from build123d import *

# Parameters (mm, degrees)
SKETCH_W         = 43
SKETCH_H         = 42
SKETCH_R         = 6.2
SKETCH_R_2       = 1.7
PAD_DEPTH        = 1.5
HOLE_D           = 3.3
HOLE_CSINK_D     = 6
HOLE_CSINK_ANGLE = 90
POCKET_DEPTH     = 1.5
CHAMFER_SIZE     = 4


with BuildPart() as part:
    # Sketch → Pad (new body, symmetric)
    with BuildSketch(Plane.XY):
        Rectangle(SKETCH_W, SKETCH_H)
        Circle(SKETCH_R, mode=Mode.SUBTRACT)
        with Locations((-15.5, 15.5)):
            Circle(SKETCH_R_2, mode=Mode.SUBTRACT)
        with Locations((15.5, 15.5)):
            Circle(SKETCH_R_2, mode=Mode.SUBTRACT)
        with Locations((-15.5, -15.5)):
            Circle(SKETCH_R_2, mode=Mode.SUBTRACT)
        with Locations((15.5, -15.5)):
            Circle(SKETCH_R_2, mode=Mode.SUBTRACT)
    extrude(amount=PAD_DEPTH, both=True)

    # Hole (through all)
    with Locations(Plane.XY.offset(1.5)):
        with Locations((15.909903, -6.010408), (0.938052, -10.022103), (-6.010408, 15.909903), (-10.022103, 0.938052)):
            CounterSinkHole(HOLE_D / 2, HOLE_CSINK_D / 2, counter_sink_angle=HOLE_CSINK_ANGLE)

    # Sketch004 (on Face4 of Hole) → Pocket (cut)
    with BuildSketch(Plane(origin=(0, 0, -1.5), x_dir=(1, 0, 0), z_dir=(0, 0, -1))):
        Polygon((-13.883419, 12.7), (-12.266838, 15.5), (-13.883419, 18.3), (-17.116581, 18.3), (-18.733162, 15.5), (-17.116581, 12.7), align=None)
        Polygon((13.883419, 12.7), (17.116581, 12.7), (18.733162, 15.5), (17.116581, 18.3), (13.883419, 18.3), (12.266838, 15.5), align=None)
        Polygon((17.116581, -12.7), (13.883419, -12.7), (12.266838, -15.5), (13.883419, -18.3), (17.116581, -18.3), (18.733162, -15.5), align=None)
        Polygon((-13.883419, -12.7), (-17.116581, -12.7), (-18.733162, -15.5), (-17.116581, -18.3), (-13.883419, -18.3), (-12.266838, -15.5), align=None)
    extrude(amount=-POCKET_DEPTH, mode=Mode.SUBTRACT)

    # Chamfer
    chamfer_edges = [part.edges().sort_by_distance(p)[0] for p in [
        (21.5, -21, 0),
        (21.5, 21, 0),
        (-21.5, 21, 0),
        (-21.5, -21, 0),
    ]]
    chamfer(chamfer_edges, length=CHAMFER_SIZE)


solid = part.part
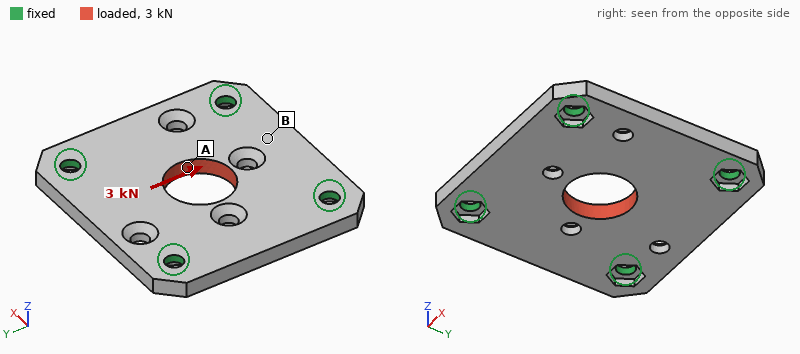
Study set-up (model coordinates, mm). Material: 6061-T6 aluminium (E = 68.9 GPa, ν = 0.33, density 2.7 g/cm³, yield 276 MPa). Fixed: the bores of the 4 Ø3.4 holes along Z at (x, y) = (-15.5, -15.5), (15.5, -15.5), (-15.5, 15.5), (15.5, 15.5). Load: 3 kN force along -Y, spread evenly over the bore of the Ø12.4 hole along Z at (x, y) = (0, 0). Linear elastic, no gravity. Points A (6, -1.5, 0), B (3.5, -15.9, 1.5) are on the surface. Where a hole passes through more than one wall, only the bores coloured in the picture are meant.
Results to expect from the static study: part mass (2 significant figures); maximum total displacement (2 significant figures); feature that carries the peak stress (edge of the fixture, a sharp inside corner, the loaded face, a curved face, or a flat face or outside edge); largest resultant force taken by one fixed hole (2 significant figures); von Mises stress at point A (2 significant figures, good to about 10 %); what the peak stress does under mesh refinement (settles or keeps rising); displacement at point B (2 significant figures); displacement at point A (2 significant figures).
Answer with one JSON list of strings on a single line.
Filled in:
["12 g", "14 µm", "edge of the fixture", "850 N", "45 MPa", "keeps rising", "7.5 µm", "9.2 µm"]
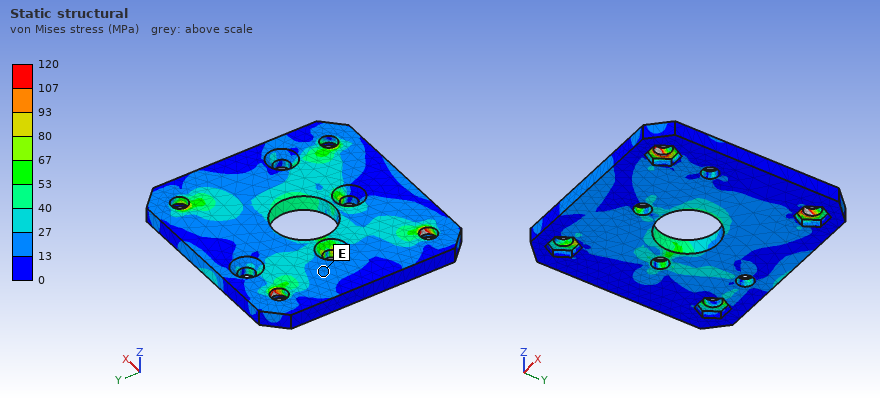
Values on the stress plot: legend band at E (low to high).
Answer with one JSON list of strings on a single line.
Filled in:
["13 to 27 MPa"]
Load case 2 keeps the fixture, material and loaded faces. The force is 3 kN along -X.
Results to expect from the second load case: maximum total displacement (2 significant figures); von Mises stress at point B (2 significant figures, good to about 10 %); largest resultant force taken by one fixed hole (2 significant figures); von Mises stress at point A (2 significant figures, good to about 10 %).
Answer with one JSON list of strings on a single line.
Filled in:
["13 µm", "17 MPa", "840 N", "27 MPa"]
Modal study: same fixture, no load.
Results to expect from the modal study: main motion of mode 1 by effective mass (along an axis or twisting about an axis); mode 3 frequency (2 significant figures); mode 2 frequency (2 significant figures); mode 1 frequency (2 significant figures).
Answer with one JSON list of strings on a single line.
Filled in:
["along Z", "14 kHz", "13 kHz", "9900 Hz"]
